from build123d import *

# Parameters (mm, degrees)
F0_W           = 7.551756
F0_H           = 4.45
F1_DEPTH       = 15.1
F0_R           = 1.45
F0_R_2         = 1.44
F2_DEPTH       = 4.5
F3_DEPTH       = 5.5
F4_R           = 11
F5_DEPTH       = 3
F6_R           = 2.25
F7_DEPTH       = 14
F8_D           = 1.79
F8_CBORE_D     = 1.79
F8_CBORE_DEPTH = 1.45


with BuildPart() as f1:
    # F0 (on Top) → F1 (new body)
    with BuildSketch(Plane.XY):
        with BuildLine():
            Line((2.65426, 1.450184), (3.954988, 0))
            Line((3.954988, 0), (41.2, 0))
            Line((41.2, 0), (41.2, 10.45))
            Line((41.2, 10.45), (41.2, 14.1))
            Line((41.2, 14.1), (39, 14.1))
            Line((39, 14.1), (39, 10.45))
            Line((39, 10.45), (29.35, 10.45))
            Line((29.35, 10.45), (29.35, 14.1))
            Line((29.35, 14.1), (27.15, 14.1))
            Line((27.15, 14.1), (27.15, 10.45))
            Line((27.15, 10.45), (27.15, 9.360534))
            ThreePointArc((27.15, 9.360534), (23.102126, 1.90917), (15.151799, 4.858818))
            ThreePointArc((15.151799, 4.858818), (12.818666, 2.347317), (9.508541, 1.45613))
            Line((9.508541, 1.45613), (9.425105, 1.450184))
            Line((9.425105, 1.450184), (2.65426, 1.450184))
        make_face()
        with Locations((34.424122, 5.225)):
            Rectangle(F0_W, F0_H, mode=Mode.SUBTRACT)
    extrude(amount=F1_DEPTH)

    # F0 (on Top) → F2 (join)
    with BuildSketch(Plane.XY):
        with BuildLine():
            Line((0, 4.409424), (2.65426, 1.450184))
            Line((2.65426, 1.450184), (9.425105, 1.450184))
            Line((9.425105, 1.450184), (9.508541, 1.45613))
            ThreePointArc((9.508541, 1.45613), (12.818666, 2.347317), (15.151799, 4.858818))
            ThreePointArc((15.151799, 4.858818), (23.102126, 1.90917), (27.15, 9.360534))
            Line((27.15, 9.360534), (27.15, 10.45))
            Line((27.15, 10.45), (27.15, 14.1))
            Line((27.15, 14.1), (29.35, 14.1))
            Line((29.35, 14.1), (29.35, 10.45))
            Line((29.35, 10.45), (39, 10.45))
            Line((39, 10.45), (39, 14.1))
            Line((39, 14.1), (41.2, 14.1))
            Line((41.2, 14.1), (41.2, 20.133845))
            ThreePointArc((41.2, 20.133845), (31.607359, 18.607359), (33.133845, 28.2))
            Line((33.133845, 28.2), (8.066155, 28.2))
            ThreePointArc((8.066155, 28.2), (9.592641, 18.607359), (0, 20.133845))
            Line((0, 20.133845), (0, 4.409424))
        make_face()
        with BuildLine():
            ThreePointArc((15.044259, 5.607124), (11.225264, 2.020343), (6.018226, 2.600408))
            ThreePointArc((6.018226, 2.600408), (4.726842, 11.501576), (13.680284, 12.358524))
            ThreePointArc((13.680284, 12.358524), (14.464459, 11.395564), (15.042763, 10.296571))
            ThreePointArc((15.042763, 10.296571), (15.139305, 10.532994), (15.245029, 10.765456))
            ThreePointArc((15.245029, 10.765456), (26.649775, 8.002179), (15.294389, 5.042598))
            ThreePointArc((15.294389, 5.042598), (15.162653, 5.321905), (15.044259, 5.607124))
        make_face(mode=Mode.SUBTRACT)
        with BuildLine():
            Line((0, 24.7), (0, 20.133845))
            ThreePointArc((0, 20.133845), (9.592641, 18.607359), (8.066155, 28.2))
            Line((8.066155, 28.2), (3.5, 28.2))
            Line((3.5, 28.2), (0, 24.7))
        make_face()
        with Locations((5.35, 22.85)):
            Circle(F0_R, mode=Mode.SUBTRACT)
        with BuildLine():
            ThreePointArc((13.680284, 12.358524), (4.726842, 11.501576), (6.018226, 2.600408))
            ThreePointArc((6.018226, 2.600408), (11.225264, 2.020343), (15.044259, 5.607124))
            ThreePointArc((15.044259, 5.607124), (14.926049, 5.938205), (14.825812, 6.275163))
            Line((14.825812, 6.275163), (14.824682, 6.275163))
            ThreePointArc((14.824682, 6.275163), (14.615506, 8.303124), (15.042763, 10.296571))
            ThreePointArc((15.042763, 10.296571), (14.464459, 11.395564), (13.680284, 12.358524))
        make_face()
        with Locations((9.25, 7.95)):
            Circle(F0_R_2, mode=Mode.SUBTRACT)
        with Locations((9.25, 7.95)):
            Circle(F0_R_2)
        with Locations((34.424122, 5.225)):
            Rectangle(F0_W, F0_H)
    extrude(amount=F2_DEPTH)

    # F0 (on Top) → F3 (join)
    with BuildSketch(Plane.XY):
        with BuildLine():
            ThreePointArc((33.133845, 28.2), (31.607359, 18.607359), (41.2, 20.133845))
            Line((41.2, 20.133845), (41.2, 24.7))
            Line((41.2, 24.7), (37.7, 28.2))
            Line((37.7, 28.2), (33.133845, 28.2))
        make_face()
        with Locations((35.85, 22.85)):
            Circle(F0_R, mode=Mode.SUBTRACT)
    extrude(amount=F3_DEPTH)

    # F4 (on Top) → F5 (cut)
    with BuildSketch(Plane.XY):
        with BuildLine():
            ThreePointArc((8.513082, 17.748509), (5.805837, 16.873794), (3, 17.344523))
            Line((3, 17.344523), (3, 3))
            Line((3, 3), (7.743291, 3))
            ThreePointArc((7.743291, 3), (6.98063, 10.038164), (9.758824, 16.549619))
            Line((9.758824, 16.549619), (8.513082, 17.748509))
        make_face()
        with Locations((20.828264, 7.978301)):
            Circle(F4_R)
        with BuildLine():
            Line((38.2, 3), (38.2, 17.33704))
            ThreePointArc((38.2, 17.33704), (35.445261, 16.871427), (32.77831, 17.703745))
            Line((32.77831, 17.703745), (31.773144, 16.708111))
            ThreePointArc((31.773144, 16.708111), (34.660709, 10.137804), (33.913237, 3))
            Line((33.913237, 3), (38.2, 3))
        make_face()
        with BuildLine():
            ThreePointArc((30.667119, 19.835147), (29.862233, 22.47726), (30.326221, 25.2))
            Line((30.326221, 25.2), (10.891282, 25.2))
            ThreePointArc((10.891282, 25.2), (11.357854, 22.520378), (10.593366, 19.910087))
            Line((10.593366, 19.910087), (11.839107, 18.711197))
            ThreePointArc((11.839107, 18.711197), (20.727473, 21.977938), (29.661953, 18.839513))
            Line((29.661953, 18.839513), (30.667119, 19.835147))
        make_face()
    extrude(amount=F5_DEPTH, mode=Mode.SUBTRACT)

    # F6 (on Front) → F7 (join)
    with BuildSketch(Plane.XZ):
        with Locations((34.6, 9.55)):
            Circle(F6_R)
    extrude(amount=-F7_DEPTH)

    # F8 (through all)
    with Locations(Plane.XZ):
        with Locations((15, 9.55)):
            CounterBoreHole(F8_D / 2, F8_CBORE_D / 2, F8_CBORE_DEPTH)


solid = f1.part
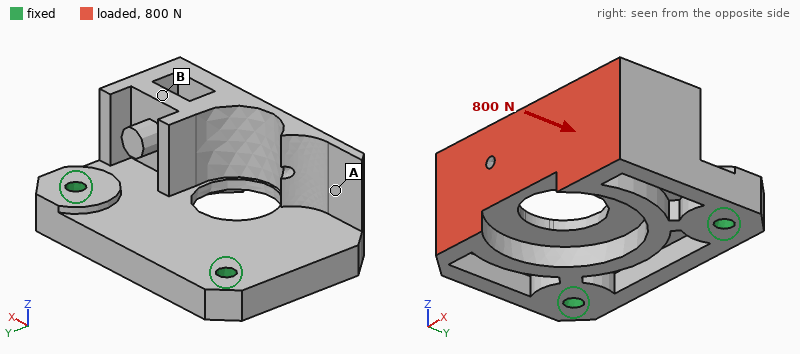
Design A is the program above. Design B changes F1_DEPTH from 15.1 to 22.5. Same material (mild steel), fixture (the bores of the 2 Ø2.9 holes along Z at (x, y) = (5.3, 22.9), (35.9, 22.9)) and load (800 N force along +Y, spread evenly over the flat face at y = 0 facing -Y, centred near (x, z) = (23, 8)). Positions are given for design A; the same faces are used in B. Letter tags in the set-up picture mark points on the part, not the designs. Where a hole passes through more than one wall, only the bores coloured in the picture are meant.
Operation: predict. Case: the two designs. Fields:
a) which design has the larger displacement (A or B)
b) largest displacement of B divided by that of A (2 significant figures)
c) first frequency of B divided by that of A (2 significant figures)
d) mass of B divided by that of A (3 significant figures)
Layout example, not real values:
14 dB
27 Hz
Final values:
B
2.2
0.70
1.25
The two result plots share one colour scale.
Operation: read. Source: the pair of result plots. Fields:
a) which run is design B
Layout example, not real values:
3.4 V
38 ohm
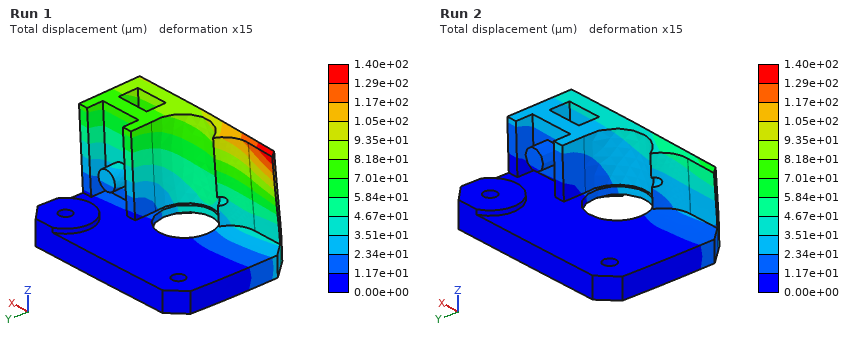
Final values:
Run 1
